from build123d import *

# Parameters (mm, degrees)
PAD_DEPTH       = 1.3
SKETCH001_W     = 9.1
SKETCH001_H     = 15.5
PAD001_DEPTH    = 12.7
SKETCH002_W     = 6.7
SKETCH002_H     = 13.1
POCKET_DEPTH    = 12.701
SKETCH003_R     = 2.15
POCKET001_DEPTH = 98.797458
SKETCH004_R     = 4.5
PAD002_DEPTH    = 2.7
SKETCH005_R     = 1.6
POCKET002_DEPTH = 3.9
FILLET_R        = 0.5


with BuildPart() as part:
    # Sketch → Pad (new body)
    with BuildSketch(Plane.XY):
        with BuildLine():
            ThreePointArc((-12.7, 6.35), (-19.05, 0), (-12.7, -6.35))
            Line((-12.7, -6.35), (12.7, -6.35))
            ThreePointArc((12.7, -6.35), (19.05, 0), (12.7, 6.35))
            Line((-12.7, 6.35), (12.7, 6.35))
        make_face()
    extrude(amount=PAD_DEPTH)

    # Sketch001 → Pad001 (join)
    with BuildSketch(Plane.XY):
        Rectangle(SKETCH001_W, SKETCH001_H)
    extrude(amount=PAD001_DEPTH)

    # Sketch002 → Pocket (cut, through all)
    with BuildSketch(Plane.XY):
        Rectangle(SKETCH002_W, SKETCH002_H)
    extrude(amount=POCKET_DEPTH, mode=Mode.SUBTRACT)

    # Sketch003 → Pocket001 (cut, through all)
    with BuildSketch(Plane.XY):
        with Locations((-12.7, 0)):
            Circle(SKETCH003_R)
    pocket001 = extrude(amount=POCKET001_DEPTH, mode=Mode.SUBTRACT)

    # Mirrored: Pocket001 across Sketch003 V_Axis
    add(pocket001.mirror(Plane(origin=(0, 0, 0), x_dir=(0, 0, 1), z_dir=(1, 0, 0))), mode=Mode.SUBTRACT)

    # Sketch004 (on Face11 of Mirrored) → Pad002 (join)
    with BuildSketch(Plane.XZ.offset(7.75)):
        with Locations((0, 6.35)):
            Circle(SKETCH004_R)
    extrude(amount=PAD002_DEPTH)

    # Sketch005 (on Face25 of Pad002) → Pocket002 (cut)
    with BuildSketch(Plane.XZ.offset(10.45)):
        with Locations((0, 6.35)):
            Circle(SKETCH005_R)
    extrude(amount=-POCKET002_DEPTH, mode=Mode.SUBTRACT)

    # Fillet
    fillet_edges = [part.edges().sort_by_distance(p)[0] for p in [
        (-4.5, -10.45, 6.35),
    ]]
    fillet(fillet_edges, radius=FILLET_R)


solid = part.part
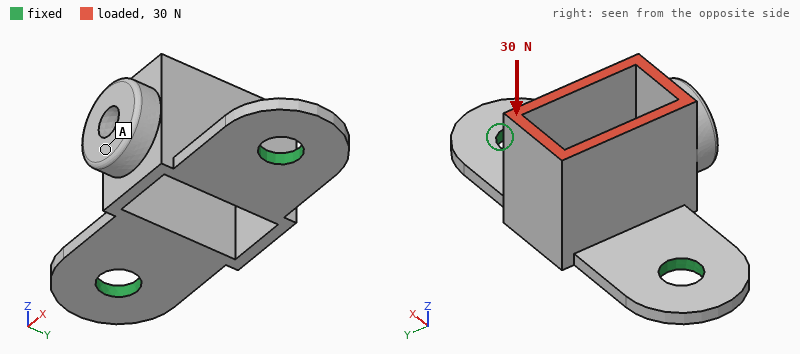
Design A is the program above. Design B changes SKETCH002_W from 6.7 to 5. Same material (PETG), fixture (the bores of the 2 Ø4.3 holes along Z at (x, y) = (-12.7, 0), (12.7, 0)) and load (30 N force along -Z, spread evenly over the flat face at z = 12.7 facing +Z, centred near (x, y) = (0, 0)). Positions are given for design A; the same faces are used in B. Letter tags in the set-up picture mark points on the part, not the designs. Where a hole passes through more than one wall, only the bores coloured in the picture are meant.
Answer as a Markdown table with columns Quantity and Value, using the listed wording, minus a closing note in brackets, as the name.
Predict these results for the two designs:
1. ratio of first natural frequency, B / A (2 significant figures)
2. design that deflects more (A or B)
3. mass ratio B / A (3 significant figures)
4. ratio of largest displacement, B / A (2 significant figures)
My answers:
| Quantity | Value |
|---|---|
| ratio of first natural frequency, B / A | 0.92 |
| design that deflects more | A |
| mass ratio B / A | 1.23 |
| ratio of largest displacement, B / A | 0.79 |
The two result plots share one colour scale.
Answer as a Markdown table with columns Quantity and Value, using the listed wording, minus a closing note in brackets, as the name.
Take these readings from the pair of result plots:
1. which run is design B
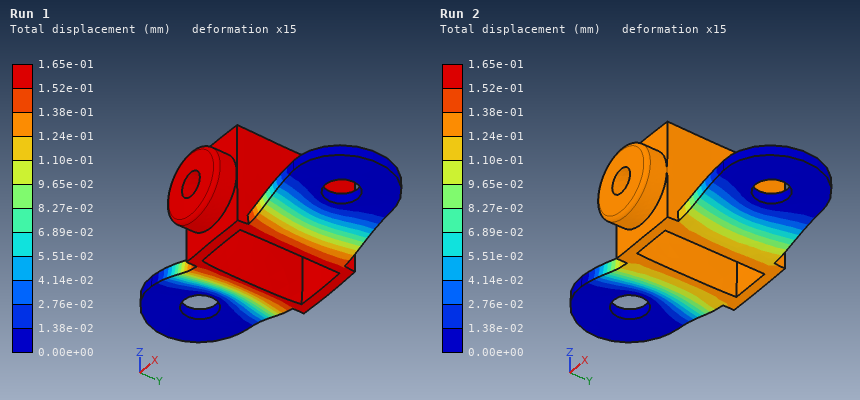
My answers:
| Quantity | Value |
|---|---|
| which run is design B | Run 2 |
